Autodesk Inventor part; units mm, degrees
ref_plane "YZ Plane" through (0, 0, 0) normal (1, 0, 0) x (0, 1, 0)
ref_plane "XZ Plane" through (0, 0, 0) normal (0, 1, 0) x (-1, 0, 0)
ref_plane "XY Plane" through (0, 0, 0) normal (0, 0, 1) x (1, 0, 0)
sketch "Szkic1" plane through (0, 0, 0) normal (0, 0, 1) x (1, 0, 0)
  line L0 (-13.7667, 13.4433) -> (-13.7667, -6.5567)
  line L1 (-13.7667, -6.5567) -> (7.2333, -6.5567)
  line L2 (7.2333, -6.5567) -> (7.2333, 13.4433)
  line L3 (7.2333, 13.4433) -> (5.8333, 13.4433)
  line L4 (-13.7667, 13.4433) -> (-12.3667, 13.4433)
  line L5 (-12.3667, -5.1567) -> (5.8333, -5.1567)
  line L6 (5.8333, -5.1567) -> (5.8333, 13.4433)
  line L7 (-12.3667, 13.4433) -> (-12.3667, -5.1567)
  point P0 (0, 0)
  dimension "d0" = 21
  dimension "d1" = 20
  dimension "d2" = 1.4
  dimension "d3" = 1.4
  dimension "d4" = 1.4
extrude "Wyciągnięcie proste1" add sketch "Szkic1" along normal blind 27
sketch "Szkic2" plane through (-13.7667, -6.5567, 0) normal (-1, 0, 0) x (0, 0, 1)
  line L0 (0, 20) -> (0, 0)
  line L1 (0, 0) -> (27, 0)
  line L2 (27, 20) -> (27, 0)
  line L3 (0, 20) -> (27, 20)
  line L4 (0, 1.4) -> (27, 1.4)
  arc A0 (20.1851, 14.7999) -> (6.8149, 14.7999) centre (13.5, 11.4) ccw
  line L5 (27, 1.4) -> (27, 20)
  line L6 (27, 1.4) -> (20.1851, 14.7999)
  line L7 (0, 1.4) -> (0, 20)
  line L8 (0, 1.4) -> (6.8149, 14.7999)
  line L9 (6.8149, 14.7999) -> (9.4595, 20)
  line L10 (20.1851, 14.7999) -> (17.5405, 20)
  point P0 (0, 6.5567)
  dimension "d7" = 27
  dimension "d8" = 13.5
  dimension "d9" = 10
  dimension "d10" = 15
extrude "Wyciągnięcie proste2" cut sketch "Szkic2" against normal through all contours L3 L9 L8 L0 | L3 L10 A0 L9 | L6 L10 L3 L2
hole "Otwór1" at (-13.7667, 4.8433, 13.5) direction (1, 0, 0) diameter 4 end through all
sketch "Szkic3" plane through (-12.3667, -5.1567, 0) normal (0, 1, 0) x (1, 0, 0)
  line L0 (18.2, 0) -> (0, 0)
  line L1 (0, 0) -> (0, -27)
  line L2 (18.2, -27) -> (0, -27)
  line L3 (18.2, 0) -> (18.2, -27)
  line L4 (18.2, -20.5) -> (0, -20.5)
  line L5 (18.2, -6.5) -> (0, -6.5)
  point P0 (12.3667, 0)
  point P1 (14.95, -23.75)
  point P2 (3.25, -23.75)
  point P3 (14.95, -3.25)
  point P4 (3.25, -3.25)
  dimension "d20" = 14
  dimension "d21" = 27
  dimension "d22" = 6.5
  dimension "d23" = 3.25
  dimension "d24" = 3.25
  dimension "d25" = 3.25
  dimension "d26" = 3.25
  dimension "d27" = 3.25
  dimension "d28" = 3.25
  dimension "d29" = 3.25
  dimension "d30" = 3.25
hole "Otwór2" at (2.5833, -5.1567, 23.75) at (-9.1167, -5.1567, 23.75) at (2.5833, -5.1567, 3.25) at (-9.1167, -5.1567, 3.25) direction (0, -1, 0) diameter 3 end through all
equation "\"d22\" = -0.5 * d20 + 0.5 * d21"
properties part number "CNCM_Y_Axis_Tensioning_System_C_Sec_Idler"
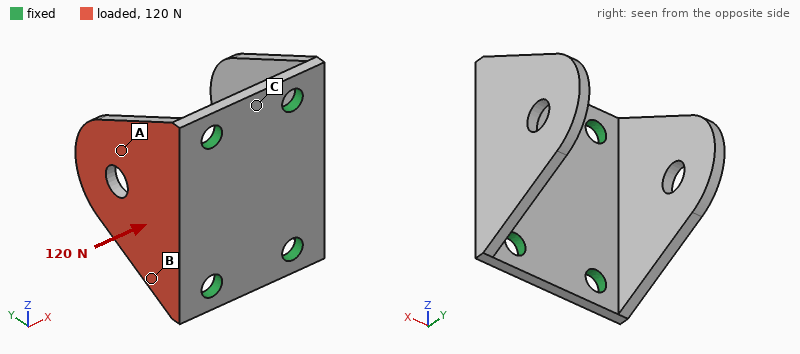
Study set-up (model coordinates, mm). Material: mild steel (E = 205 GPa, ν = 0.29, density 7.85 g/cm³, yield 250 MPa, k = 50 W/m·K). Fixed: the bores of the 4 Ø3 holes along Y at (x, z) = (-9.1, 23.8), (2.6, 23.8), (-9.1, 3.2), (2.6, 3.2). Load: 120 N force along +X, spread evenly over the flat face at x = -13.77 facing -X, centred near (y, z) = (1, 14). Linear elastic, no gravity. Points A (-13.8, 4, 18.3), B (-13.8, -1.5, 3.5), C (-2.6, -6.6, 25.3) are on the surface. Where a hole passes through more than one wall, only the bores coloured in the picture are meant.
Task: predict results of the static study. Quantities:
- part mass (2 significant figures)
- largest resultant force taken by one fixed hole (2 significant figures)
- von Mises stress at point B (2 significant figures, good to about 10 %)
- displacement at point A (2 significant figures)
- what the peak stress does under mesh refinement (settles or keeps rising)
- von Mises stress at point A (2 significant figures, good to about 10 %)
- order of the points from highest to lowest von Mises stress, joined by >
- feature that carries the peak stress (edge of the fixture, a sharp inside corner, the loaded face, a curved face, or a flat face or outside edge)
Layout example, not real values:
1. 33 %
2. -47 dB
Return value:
1. 12 g
2. 43 N
3. 65 MPa
4. 42 µm
5. keeps rising
6. 29 MPa
7. B > A > C
8. edge of the fixture
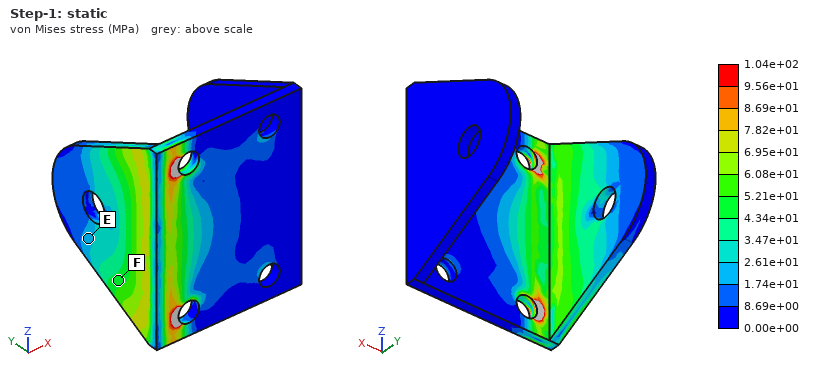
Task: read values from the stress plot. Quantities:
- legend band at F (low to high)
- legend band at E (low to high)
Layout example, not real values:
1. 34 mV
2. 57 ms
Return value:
1. 4.34e+01 to 5.21e+01 MPa
2. 1.74e+01 to 2.61e+01 MPa
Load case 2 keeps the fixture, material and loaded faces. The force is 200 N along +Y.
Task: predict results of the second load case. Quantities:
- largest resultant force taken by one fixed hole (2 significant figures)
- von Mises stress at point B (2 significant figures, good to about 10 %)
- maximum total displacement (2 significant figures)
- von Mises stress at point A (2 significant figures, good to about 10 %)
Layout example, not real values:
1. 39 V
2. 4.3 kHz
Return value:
1. 110 N
2. 19 MPa
3. 35 µm
4. 11 MPa
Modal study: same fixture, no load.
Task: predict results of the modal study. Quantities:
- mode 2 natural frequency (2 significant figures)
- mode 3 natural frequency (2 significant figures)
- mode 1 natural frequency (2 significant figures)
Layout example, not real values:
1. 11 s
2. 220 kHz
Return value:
1. 4000 Hz
2. 12 kHz
3. 3900 Hz
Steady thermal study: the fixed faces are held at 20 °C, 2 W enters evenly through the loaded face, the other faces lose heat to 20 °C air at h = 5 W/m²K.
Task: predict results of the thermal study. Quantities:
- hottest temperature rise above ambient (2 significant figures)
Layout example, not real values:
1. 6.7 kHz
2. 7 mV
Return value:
1. 15 K
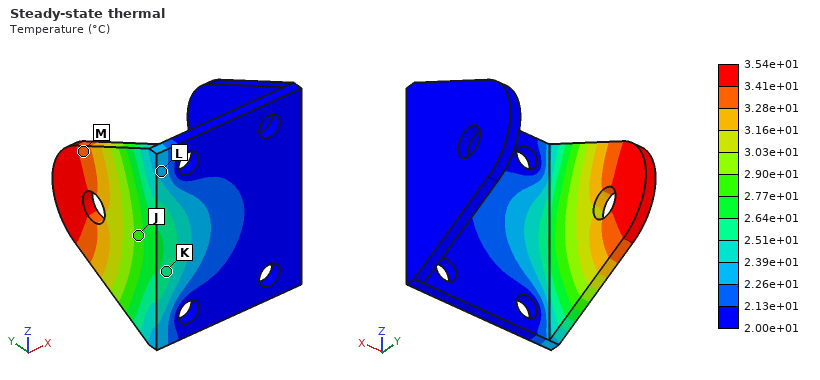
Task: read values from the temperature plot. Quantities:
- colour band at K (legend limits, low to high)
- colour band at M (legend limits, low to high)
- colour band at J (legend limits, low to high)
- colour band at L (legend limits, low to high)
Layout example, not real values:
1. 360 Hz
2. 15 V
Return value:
1. 2.51e+01 to 2.64e+01 °C
2. 3.28e+01 to 3.41e+01 °C
3. 2.77e+01 to 2.90e+01 °C
4. 2.26e+01 to 2.39e+01 °C
